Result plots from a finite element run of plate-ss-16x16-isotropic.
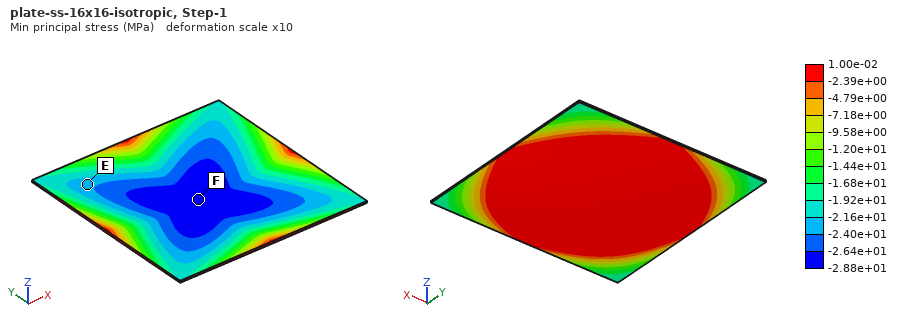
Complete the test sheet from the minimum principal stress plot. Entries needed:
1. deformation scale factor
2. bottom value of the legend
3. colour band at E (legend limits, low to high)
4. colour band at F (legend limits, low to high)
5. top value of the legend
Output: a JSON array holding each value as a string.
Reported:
["10", "-2.88e+01 MPa", "-2.40e+01 to -2.16e+01 MPa", "-2.88e+01 to -2.64e+01 MPa", "1.00e-02 MPa"]
